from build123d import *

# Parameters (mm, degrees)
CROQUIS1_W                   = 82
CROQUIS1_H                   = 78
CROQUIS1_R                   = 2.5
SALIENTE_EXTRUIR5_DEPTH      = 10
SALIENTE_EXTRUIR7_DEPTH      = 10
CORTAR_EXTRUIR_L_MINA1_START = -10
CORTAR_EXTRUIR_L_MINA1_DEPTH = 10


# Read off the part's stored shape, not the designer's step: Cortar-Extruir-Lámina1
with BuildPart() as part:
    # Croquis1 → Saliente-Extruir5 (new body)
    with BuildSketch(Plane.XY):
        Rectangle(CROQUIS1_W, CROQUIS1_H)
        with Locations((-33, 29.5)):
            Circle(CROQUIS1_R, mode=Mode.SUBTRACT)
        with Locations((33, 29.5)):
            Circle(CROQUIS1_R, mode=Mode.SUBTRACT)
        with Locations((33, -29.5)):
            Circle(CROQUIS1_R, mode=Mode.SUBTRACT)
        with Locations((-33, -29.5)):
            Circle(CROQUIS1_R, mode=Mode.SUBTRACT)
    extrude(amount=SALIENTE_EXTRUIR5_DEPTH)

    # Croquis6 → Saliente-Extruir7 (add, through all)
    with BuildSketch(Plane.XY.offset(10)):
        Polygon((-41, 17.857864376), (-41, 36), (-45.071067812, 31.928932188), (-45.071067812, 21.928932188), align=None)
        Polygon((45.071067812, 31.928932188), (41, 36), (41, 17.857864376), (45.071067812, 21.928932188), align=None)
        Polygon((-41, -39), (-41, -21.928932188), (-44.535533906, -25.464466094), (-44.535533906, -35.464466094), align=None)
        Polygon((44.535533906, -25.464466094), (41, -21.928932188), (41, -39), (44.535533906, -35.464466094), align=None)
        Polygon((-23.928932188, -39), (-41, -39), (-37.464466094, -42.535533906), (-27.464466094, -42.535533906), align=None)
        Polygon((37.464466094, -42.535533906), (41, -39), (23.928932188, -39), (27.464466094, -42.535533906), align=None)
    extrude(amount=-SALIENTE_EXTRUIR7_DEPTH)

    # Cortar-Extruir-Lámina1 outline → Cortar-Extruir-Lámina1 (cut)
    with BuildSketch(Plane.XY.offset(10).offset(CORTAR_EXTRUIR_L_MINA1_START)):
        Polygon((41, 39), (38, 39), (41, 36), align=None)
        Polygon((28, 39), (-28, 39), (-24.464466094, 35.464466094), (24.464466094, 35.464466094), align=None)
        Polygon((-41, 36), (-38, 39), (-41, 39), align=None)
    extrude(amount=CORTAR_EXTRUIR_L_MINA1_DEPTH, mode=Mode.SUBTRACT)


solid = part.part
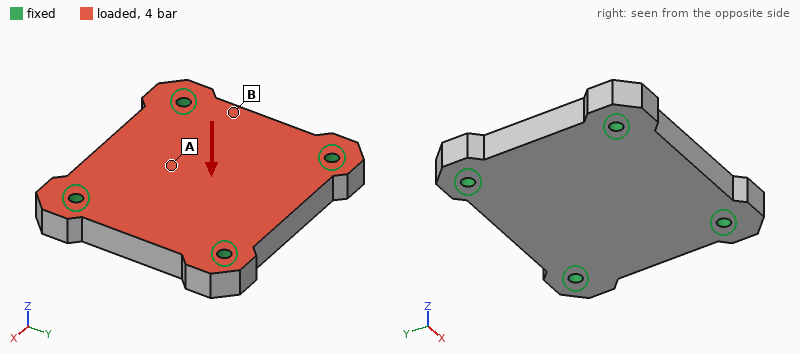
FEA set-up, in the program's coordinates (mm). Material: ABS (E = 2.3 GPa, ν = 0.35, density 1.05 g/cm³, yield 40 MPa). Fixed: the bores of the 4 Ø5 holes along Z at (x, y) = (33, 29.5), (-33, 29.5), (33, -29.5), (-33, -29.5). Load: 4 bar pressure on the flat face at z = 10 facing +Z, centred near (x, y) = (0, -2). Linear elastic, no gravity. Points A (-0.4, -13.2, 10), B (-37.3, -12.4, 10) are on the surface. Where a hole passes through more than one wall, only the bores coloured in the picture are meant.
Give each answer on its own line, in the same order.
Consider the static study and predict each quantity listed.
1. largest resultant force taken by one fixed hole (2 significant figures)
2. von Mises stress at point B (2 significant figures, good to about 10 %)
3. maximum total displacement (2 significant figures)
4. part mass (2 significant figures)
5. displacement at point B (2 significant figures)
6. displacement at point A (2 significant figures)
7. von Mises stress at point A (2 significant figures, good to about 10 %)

670 N
2.2 MPa
0.26 mm
68 g
0.082 mm
0.24 mm
4.7 MPa
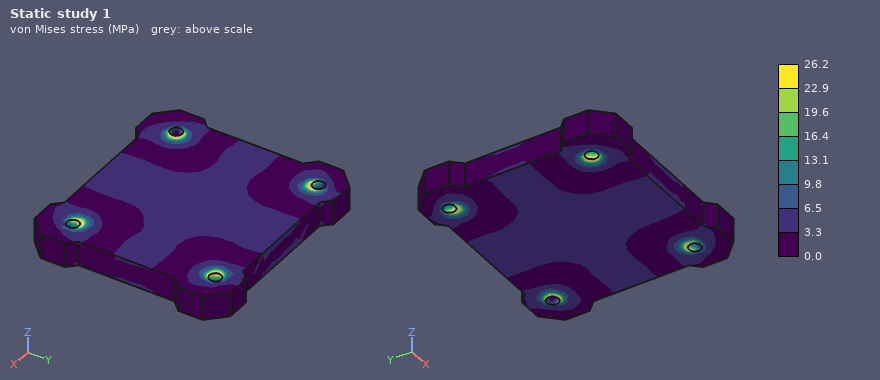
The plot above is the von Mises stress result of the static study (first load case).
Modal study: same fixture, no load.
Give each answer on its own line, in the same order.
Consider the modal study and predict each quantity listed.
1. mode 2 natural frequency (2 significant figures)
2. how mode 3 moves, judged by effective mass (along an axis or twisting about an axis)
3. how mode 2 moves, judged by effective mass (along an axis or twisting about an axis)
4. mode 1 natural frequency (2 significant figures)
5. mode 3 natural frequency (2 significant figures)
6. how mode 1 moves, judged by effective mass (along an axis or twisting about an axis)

3400 Hz
twisting about Y
twisting about X
2300 Hz
3900 Hz
along Z
